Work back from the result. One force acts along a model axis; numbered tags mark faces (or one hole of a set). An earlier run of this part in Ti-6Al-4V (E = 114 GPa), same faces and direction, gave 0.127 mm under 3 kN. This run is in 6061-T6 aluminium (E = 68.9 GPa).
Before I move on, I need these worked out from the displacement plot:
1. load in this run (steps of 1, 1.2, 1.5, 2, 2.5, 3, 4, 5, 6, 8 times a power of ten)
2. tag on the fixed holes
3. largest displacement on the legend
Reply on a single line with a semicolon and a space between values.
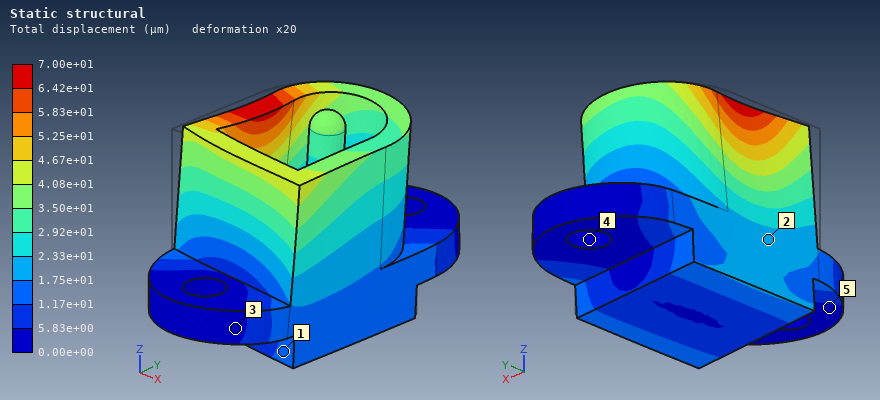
1 kN; 4; 7.00e+01 µm
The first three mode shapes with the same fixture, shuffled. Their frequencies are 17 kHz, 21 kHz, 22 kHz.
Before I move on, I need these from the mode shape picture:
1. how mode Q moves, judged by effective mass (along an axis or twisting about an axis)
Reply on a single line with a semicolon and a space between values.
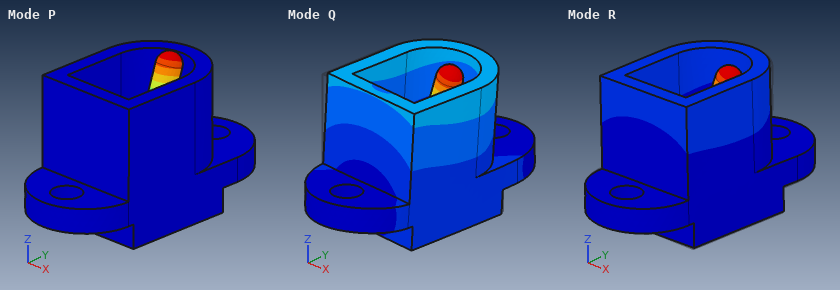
along X
